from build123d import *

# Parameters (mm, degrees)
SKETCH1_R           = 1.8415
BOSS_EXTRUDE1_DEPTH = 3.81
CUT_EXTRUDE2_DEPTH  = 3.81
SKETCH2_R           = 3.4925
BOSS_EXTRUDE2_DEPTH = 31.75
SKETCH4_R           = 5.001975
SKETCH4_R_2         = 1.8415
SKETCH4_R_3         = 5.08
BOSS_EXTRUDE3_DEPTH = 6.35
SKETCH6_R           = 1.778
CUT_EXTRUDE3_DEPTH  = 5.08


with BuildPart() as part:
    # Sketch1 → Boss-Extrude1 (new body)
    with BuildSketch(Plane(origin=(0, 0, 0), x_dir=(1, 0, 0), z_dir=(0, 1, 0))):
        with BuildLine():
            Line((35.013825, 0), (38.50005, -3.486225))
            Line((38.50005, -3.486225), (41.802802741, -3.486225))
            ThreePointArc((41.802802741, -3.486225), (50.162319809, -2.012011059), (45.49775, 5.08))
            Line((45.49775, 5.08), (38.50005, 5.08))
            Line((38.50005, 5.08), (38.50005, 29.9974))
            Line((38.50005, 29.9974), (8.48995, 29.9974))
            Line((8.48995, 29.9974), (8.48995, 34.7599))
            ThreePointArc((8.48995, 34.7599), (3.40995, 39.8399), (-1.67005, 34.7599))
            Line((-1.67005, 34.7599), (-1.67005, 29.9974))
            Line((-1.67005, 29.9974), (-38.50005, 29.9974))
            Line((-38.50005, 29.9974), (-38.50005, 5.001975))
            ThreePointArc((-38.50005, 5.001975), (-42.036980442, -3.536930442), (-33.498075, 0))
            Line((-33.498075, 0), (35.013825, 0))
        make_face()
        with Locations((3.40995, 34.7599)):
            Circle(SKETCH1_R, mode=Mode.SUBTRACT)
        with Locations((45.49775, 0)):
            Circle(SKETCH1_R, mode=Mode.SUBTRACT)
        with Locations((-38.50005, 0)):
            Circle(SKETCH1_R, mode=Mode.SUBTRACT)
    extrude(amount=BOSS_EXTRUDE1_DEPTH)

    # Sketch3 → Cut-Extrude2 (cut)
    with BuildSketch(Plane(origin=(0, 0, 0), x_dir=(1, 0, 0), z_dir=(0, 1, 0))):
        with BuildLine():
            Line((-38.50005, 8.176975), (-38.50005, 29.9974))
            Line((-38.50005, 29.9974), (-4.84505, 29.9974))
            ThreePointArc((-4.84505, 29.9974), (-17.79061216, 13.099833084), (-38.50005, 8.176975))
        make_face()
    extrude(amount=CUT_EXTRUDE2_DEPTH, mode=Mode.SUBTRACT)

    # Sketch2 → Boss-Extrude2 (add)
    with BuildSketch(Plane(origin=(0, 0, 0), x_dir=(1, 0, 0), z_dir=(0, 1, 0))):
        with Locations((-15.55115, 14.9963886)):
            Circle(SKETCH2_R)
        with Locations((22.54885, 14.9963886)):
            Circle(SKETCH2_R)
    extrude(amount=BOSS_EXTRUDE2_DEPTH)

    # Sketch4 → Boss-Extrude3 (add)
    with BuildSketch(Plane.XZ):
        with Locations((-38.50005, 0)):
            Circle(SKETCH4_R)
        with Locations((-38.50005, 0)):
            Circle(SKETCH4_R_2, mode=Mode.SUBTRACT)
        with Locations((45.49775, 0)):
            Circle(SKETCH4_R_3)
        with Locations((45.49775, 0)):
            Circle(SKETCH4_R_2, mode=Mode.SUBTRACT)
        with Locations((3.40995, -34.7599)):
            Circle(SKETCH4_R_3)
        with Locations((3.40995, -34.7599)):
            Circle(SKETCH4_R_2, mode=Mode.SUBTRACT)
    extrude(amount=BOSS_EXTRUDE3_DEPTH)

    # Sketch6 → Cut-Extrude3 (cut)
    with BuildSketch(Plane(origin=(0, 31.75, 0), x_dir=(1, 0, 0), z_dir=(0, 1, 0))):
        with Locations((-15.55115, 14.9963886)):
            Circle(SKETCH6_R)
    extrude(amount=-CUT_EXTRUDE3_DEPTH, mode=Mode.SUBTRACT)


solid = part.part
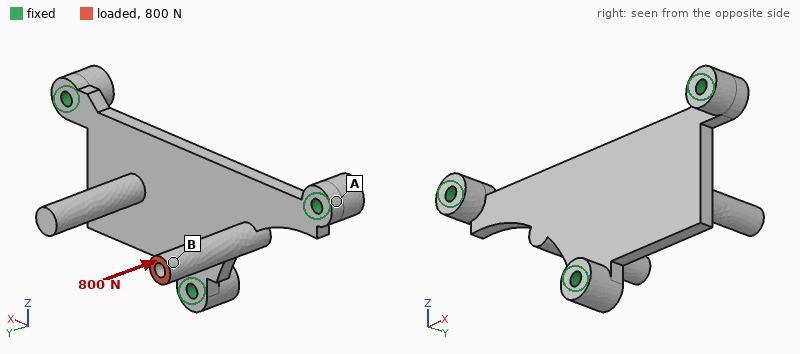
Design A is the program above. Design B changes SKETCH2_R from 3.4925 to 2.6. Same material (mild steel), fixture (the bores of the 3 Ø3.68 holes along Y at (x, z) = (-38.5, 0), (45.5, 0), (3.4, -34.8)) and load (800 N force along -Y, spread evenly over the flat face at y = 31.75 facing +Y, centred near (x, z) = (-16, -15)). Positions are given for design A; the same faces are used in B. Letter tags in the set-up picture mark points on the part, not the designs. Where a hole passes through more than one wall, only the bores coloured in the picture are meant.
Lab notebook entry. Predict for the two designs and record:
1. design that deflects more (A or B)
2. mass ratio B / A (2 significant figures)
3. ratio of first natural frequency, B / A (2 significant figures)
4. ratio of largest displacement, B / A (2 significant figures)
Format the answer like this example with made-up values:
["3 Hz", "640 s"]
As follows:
["B", "0.91", "1.1", "1.2"]
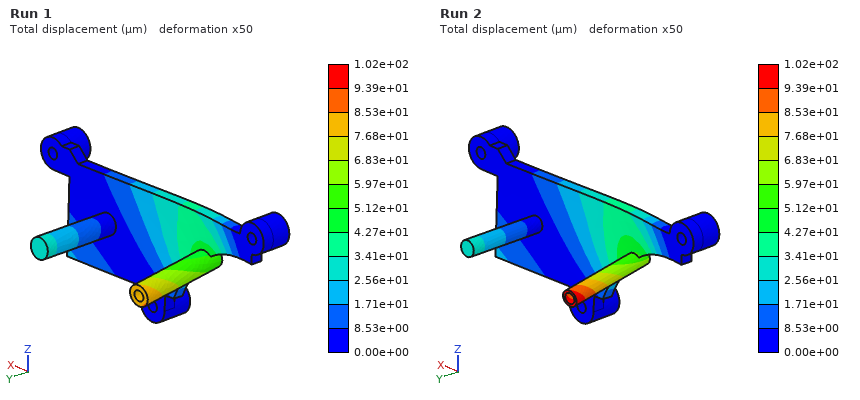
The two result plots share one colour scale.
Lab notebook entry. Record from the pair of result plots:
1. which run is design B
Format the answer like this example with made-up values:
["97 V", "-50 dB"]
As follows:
["Run 2"]
